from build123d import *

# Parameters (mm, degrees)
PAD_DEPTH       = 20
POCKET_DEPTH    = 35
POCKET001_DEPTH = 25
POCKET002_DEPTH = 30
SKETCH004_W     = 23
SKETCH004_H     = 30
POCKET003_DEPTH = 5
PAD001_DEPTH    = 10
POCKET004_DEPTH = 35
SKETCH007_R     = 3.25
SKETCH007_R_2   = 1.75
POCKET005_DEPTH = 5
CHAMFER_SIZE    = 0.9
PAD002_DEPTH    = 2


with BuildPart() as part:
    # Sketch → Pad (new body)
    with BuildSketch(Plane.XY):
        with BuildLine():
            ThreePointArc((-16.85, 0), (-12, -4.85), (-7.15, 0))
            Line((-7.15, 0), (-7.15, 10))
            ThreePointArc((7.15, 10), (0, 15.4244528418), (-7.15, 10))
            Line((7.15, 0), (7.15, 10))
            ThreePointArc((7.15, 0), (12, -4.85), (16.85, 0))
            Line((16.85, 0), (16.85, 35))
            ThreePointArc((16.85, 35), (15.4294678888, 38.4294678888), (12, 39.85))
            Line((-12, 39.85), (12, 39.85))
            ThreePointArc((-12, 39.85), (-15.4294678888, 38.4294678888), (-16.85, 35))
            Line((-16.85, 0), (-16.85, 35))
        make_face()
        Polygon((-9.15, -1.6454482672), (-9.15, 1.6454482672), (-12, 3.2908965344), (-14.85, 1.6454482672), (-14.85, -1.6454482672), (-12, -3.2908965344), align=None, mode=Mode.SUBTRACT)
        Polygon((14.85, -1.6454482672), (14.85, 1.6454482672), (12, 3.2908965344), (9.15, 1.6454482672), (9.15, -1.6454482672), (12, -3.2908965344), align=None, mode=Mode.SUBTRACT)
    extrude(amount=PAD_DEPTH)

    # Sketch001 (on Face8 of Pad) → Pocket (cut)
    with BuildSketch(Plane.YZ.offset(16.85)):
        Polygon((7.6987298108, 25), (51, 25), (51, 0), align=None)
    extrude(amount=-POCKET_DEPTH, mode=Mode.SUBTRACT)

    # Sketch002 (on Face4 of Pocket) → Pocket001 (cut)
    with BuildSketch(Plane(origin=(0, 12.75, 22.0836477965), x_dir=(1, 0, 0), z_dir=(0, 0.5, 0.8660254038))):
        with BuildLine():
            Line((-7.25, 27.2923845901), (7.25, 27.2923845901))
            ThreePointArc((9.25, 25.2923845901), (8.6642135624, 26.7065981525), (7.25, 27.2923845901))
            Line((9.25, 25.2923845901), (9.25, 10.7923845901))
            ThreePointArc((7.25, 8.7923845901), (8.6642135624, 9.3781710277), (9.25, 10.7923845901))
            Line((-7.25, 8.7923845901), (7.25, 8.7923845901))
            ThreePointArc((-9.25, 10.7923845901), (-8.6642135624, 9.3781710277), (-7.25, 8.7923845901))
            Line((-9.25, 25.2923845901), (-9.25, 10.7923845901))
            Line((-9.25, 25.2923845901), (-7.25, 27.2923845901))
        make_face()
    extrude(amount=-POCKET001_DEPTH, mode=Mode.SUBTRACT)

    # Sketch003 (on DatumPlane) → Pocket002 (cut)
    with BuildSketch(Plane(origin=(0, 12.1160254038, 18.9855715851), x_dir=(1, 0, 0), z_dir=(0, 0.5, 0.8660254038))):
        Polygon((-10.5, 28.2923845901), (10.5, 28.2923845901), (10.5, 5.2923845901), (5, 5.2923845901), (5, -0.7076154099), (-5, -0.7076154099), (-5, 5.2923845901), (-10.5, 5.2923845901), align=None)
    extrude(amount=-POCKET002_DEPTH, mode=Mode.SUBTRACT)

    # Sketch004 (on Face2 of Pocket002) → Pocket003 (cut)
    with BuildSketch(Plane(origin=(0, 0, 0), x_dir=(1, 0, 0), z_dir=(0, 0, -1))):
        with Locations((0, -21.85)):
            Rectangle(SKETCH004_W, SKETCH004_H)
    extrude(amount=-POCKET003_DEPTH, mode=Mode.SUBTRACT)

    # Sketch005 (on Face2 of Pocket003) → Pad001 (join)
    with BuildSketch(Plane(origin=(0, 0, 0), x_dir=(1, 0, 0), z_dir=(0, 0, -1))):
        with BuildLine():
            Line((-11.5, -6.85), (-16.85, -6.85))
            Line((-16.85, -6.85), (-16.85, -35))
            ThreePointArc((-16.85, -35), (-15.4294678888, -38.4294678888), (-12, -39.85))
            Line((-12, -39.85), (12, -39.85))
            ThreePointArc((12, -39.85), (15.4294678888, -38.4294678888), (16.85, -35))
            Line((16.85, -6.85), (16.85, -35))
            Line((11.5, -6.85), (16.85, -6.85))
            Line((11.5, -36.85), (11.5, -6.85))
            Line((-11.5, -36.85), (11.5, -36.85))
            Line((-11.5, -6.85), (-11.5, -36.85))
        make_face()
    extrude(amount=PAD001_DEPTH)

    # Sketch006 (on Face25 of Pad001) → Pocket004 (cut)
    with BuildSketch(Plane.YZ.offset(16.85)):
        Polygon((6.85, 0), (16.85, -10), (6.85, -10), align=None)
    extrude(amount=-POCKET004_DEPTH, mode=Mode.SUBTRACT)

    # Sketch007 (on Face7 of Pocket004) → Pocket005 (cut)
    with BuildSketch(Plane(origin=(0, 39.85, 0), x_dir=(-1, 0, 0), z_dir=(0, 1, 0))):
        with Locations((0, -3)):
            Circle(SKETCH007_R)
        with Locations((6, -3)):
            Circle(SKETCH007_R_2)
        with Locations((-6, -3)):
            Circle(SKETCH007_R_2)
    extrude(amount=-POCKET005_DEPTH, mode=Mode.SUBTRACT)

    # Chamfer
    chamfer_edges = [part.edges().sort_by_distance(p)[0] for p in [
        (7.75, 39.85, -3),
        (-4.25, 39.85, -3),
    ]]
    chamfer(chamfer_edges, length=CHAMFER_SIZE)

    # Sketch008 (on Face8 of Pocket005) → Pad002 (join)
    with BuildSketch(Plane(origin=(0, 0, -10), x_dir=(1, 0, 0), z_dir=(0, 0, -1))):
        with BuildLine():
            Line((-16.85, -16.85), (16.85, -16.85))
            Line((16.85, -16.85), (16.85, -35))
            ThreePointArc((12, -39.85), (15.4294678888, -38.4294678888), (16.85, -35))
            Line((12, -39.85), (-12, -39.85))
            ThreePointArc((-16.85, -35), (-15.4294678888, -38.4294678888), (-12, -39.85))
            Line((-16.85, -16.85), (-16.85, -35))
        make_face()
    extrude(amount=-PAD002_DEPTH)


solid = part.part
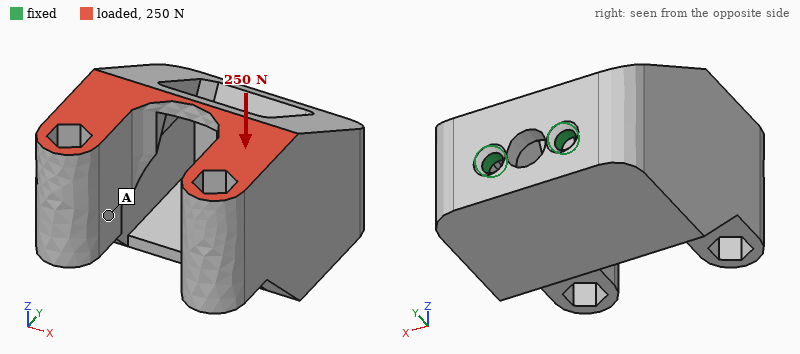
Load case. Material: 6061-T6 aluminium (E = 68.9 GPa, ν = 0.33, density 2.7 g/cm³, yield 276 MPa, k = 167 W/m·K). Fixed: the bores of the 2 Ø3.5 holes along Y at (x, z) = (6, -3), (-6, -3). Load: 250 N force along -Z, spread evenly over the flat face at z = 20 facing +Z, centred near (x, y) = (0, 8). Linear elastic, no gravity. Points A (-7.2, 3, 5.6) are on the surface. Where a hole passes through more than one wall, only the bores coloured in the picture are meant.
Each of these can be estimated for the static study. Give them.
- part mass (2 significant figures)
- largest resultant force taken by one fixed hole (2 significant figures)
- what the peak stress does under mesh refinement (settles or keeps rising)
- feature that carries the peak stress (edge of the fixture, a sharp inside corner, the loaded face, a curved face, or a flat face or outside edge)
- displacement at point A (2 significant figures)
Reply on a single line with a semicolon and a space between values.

41 g; 130 N; keeps rising; edge of the fixture; 0.16 mm
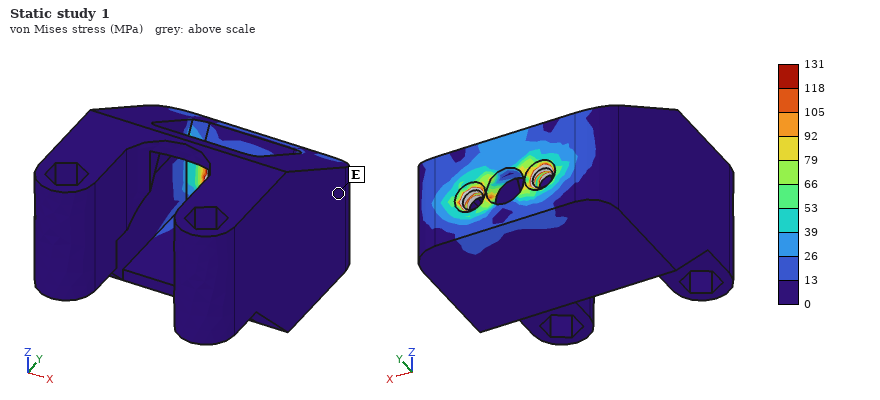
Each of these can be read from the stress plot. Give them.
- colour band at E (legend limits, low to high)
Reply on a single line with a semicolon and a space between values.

0 to 13 MPa
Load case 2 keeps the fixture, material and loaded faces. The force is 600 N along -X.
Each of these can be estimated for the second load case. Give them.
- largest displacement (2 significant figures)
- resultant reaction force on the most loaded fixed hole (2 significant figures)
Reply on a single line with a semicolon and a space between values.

0.23 mm; 1.4 kN
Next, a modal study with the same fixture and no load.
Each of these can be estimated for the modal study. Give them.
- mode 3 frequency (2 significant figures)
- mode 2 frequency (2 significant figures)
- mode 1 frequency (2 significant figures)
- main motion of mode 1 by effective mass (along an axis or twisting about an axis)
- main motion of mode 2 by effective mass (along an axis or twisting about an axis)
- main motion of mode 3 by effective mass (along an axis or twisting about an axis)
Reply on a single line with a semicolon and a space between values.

3600 Hz; 2100 Hz; 1200 Hz; along Z; along X; twisting about Y
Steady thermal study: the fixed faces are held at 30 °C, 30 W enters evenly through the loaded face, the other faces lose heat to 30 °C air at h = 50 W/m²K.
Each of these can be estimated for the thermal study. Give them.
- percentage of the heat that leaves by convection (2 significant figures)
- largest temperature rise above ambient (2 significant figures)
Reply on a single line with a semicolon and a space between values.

24 %; 29 K
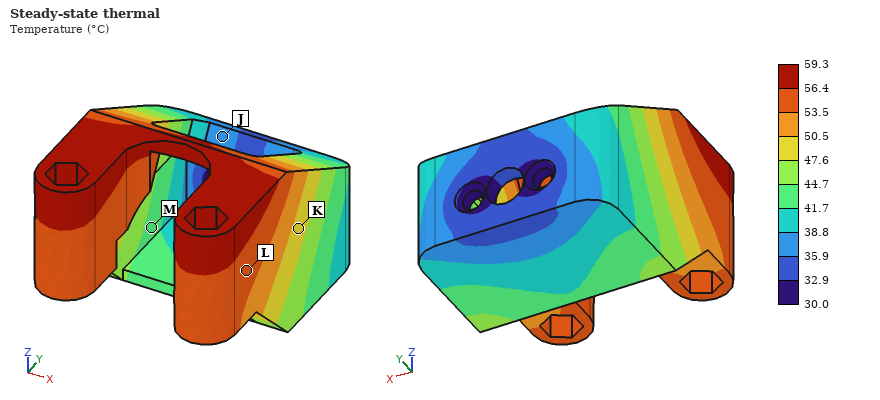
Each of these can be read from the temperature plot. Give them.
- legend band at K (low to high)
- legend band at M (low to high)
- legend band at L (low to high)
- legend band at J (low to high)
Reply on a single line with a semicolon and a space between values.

47.6 to 50.5 °C; 41.7 to 44.7 °C; 53.5 to 56.4 °C; 35.9 to 38.8 °C
